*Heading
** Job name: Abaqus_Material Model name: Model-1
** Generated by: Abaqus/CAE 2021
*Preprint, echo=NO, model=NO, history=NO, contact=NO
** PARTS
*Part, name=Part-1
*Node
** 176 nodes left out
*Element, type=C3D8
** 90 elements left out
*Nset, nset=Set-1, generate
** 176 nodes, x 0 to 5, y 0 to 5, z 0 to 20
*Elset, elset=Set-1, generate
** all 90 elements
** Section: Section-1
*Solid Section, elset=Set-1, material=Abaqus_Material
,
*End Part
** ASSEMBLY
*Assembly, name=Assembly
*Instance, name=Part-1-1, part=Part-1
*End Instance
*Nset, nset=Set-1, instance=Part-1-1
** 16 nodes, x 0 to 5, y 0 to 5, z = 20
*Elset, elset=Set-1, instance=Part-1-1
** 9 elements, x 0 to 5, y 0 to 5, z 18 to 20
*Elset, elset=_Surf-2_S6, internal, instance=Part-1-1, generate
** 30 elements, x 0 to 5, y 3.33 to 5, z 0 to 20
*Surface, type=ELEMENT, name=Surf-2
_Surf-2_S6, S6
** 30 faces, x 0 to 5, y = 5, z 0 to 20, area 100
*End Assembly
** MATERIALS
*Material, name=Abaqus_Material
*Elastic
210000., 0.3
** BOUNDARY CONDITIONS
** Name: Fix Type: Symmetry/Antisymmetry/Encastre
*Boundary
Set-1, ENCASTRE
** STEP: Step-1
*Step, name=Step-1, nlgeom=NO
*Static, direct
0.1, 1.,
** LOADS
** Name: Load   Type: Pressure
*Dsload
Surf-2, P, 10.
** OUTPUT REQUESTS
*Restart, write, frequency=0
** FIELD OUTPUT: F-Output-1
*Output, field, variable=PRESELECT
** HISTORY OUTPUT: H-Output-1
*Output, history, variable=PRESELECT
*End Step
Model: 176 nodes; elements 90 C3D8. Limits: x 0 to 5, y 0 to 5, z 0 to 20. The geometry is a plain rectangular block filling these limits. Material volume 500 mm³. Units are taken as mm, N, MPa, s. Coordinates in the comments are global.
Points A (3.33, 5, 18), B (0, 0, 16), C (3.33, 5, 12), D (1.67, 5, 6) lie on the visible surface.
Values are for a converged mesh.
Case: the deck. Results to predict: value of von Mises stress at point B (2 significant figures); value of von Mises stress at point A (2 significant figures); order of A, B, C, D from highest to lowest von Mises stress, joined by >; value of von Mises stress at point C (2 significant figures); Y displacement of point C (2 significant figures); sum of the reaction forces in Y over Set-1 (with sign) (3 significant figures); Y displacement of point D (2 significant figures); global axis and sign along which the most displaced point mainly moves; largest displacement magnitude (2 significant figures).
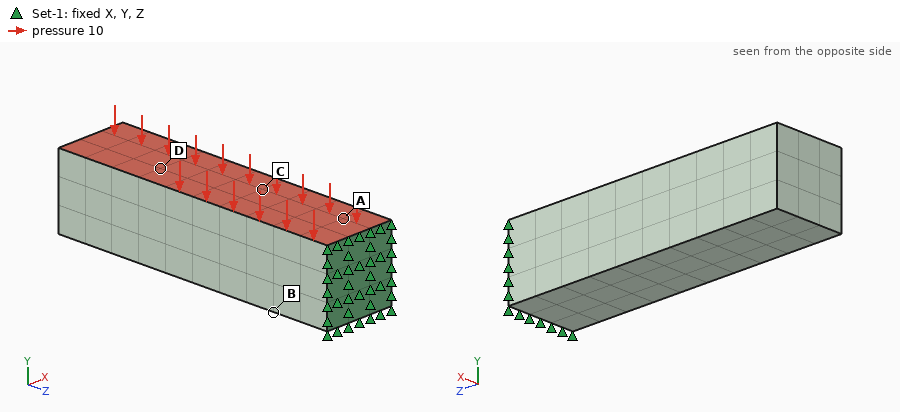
300 MPa
410 MPa
A > B > C > D
180 MPa
-0.025 mm
1000 N
-0.059 mm
-Y
0.096 mm
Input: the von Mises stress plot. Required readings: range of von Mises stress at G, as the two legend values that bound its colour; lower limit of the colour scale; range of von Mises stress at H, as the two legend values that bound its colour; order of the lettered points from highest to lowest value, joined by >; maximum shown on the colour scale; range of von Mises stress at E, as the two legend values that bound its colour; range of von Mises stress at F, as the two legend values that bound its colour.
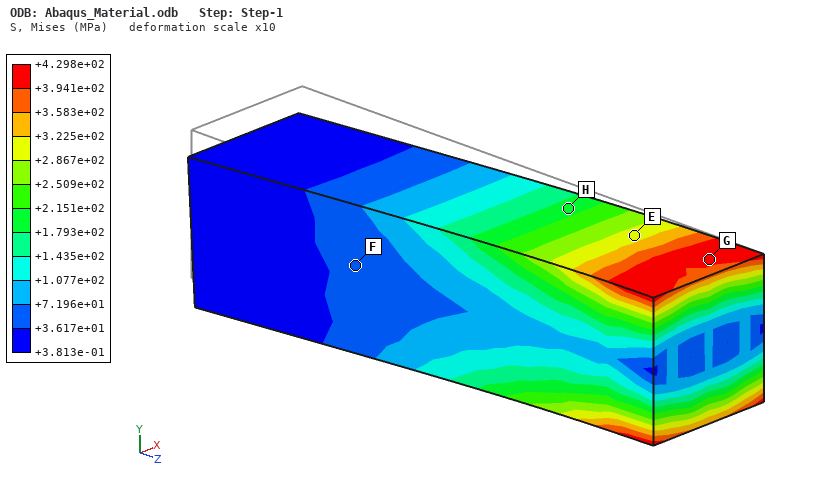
+3.941e+02 to +4.298e+02 MPa
+3.813e-01 MPa
+1.793e+02 to +2.151e+02 MPa
G > E > H > F
+4.298e+02 MPa
+2.867e+02 to +3.225e+02 MPa
+3.617e+01 to +7.196e+01 MPa
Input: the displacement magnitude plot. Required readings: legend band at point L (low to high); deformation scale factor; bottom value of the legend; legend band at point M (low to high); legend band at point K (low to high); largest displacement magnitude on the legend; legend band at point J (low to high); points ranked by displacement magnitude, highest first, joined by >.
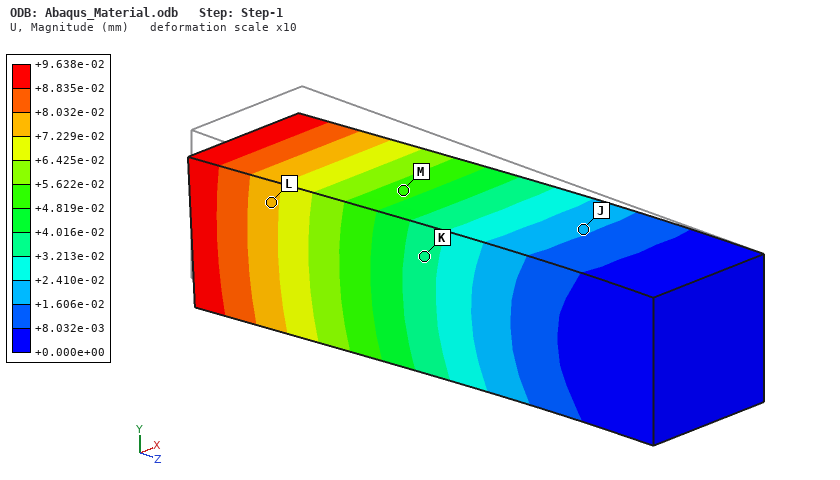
+7.229e-02 to +8.032e-02 mm
10
+0.000e+00 mm
+4.819e-02 to +5.622e-02 mm
+3.213e-02 to +4.016e-02 mm
+9.638e-02 mm
+1.606e-02 to +2.410e-02 mm
L > M > K > J
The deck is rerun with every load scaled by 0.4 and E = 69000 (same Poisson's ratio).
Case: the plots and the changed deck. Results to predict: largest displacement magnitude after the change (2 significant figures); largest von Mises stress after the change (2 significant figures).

0.12 mm
170 MPa
